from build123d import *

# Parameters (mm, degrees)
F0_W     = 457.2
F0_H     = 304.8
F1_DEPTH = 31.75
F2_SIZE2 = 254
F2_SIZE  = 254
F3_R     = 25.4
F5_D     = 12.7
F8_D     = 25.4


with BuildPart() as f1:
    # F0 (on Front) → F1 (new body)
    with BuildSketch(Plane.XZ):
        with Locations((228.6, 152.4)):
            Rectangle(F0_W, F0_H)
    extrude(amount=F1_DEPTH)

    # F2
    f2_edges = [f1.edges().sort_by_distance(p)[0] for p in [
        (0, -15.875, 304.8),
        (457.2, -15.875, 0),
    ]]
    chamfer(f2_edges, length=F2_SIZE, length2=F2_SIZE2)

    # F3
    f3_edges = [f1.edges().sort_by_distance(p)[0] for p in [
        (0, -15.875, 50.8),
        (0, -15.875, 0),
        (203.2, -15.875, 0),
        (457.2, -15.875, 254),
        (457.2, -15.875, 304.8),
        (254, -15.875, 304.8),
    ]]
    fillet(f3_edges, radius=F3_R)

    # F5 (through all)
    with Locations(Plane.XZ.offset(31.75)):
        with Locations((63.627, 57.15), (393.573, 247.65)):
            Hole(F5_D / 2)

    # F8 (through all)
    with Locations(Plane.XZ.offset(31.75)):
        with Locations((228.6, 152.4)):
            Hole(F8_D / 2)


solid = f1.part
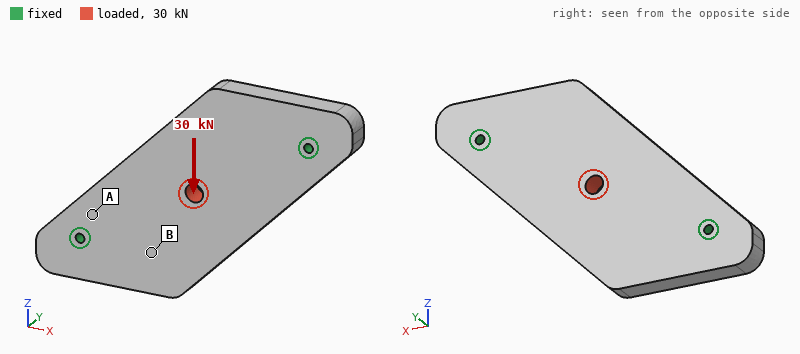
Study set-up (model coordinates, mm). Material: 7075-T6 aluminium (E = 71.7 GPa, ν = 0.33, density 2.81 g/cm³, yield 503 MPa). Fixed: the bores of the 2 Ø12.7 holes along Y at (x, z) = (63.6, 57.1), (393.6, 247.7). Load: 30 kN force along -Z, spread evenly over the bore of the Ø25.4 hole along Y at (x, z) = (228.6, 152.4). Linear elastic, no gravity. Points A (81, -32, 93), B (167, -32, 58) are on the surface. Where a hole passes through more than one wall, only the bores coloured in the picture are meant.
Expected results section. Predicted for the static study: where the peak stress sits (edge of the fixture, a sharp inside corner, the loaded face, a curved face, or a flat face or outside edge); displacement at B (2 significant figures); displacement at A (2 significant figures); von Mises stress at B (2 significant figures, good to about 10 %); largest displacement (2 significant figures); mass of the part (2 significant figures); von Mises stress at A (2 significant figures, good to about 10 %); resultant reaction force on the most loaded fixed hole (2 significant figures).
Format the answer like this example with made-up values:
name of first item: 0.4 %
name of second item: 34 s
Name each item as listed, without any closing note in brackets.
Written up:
where the peak stress sits: edge of the fixture
displacement at B: 33 µm
displacement at A: 13 µm
von Mises stress at B: 4.5 MPa
largest displacement: 51 µm
mass of the part: 6.6 kg
von Mises stress at A: 8.4 MPa
resultant reaction force on the most loaded fixed hole: 15 kN
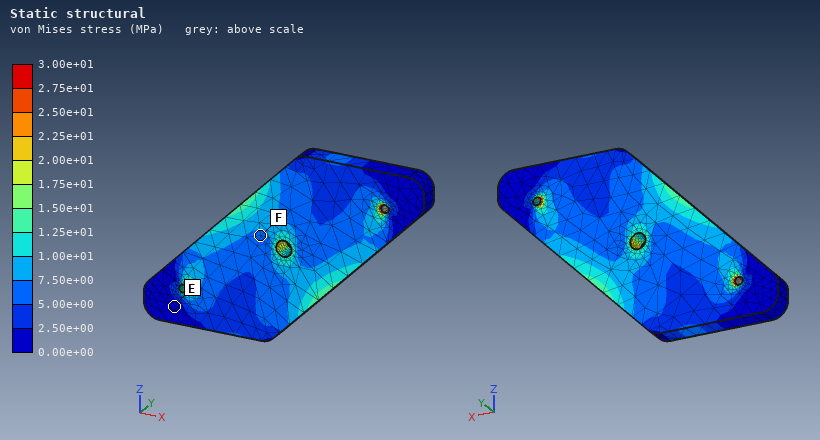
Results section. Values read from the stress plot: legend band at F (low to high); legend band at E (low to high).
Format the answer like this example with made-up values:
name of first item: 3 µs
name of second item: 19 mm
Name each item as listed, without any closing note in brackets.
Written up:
legend band at F: 5.00e+00 to 7.50e+00 MPa
legend band at E: 0.00e+00 to 2.50e+00 MPa
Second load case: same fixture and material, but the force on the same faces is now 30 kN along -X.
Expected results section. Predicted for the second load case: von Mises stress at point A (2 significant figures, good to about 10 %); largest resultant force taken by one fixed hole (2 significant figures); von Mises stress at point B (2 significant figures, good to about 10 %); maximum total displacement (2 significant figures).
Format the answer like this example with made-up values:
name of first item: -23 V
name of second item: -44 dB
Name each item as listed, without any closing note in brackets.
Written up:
von Mises stress at point A: 3.5 MPa
largest resultant force taken by one fixed hole: 15 kN
von Mises stress at point B: 4.8 MPa
maximum total displacement: 31 µm
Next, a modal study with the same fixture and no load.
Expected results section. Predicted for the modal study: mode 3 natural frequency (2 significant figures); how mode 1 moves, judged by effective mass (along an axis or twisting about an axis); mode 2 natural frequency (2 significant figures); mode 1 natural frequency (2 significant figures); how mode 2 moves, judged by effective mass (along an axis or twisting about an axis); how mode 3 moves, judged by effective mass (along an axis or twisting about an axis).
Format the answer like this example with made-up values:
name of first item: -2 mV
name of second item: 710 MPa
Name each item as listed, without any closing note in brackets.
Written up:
mode 3 natural frequency: 2100 Hz
how mode 1 moves, judged by effective mass: along Y
mode 2 natural frequency: 970 Hz
mode 1 natural frequency: 810 Hz
how mode 2 moves, judged by effective mass: twisting about X
how mode 3 moves, judged by effective mass: along Z
